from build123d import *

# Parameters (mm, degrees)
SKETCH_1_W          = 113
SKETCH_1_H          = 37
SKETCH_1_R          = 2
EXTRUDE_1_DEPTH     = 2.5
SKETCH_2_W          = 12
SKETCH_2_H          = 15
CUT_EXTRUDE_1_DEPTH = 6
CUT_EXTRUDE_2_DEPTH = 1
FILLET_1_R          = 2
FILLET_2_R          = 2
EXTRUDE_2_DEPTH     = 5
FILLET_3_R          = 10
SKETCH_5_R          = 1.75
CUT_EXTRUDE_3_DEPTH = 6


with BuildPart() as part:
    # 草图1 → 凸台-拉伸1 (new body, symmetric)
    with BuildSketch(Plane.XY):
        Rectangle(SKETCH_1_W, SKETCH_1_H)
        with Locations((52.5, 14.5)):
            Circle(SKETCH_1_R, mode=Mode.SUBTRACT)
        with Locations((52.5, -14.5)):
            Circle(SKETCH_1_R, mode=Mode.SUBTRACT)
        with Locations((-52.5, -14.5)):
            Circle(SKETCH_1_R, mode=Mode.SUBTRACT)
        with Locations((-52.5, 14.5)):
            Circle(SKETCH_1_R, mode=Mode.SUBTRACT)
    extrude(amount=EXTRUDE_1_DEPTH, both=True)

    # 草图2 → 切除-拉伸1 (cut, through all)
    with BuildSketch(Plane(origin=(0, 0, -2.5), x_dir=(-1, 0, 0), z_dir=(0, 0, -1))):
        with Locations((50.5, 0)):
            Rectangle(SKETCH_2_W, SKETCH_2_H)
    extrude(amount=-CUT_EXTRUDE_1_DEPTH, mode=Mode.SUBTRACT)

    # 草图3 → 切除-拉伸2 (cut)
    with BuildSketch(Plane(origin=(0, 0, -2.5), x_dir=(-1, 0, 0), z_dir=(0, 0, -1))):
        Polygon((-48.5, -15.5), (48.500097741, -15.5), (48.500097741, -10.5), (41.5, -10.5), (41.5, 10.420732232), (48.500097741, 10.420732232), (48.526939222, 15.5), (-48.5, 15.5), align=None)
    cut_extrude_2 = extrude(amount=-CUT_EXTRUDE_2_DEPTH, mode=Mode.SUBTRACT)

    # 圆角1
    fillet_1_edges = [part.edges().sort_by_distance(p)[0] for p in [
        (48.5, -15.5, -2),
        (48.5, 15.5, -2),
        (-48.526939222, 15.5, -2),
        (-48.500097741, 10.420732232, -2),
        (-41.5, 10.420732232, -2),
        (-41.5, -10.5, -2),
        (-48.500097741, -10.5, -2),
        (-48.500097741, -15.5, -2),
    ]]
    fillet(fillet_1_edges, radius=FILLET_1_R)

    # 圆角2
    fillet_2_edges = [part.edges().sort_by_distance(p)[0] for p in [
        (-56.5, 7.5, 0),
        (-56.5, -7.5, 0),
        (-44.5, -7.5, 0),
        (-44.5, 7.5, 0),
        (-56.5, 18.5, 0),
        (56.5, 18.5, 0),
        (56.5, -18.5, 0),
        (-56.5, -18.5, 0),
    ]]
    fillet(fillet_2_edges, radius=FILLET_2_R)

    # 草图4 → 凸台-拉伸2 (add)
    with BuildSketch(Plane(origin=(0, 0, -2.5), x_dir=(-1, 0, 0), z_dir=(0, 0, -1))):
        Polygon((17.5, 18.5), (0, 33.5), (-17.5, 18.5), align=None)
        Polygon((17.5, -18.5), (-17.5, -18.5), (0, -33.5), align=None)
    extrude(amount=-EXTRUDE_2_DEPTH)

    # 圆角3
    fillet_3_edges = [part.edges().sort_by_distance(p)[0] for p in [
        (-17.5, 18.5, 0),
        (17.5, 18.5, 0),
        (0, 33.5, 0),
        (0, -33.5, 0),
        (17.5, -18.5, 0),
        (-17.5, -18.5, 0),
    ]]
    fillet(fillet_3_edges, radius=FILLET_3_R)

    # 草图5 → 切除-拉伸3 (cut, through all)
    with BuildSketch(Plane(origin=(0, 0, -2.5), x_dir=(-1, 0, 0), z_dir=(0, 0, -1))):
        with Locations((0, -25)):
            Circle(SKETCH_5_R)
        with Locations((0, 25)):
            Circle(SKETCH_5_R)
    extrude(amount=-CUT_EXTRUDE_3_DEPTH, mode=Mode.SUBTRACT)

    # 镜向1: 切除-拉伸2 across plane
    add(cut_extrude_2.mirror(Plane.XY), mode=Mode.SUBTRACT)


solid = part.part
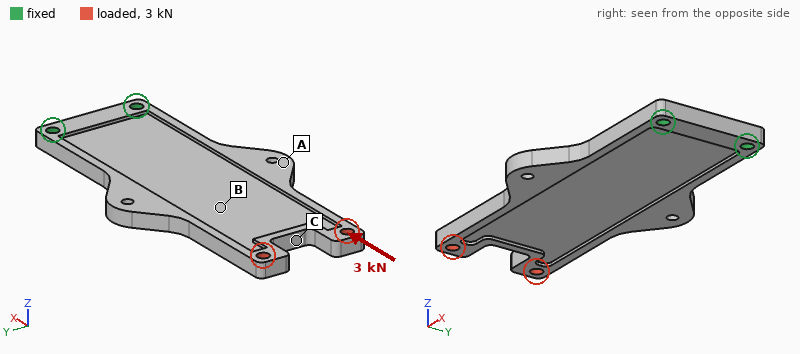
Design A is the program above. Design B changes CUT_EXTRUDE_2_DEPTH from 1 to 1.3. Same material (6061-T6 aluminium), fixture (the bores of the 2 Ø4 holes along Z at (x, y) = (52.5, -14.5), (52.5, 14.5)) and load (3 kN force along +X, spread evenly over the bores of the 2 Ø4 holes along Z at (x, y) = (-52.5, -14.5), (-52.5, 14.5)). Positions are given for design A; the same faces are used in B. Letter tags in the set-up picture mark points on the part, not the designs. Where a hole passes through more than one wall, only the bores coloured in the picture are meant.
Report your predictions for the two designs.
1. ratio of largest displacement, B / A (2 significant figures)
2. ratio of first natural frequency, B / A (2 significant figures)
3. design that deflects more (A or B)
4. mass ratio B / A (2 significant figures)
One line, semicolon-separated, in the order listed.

1.1; 0.92; B; 0.90
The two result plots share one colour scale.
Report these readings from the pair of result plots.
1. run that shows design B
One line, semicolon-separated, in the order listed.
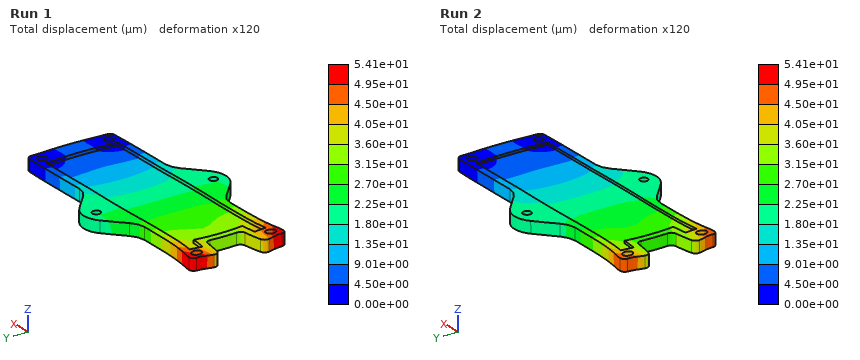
Run 1
